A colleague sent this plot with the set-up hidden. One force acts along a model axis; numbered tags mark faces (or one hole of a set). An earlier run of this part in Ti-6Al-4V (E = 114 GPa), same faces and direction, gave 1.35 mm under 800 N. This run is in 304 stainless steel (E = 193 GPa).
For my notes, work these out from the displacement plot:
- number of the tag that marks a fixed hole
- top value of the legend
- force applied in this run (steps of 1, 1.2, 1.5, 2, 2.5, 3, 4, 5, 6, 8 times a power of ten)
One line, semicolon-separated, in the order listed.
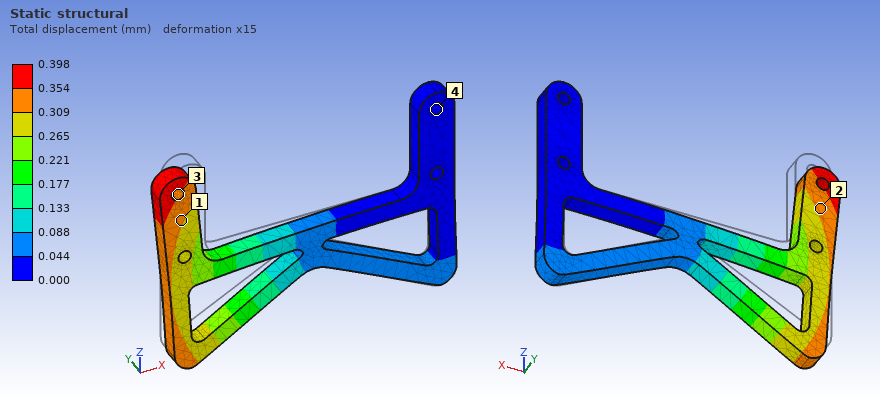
4; 0.398 mm; 400 N
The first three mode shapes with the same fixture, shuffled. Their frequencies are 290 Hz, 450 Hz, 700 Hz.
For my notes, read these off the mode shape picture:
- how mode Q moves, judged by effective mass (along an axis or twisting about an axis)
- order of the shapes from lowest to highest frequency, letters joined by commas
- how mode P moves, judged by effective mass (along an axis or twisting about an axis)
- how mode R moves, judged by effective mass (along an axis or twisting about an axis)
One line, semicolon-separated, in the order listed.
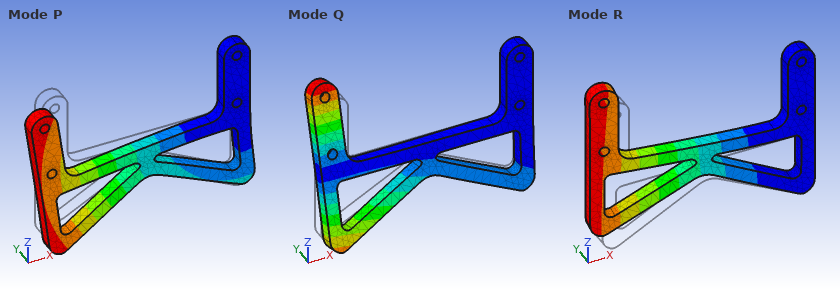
twisting about X; R, P, Q; along Z; along Y
